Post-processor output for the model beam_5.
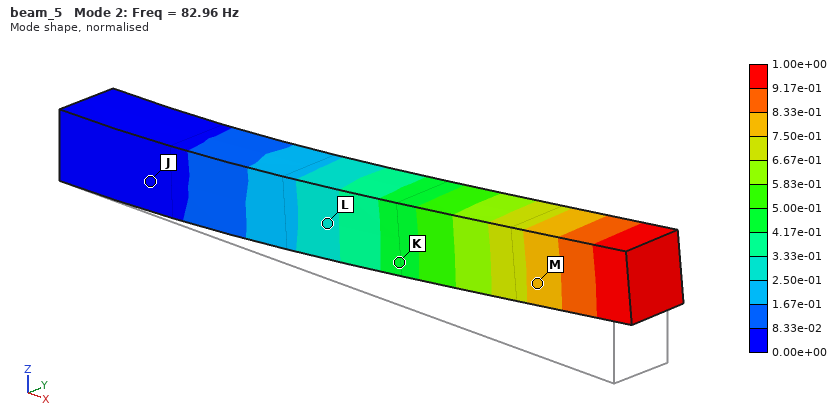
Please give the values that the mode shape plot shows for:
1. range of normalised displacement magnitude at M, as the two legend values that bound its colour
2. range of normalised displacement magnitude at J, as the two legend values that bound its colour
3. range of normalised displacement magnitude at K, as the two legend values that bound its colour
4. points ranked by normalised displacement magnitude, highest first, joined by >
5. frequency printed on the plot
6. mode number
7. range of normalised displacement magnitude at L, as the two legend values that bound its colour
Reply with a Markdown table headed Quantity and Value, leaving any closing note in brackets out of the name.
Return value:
| Quantity | Value |
|---|---|
| range of normalised displacement magnitude at M, as the two legend values that bound its colour | 7.50e-01 to 8.33e-01 |
| range of normalised displacement magnitude at J, as the two legend values that bound its colour | 0.00e+00 to 8.33e-02 |
| range of normalised displacement magnitude at K, as the two legend values that bound its colour | 4.17e-01 to 5.00e-01 |
| points ranked by normalised displacement magnitude, highest first, joined by > | M > K > L > J |
| frequency printed on the plot | 82.96 Hz |
| mode number | 2 |
| range of normalised displacement magnitude at L, as the two legend values that bound its colour | 2.50e-01 to 3.33e-01 |
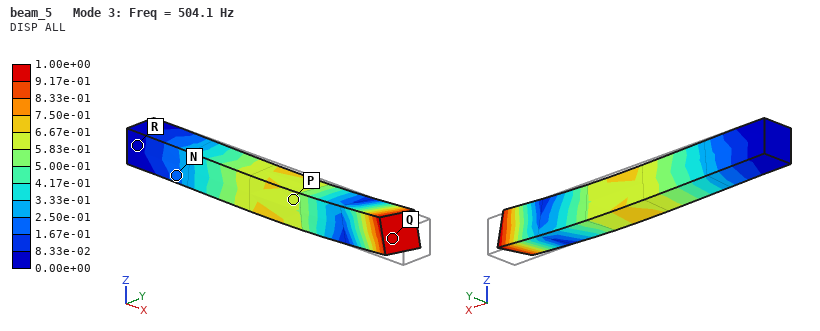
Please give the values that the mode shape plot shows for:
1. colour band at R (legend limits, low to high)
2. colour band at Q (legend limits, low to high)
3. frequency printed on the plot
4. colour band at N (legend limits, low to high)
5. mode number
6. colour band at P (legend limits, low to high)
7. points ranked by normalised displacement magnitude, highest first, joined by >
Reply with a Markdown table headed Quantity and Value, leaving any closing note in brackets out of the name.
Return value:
| Quantity | Value |
|---|---|
| colour band at R | 0.00e+00 to 8.33e-02 |
| colour band at Q | 9.17e-01 to 1.00e+00 |
| frequency printed on the plot | 504.1 Hz |
| colour band at N | 1.67e-01 to 2.50e-01 |
| mode number | 3 |
| colour band at P | 5.83e-01 to 6.67e-01 |
| points ranked by normalised displacement magnitude, highest first, joined by > | Q > P > N > R |
